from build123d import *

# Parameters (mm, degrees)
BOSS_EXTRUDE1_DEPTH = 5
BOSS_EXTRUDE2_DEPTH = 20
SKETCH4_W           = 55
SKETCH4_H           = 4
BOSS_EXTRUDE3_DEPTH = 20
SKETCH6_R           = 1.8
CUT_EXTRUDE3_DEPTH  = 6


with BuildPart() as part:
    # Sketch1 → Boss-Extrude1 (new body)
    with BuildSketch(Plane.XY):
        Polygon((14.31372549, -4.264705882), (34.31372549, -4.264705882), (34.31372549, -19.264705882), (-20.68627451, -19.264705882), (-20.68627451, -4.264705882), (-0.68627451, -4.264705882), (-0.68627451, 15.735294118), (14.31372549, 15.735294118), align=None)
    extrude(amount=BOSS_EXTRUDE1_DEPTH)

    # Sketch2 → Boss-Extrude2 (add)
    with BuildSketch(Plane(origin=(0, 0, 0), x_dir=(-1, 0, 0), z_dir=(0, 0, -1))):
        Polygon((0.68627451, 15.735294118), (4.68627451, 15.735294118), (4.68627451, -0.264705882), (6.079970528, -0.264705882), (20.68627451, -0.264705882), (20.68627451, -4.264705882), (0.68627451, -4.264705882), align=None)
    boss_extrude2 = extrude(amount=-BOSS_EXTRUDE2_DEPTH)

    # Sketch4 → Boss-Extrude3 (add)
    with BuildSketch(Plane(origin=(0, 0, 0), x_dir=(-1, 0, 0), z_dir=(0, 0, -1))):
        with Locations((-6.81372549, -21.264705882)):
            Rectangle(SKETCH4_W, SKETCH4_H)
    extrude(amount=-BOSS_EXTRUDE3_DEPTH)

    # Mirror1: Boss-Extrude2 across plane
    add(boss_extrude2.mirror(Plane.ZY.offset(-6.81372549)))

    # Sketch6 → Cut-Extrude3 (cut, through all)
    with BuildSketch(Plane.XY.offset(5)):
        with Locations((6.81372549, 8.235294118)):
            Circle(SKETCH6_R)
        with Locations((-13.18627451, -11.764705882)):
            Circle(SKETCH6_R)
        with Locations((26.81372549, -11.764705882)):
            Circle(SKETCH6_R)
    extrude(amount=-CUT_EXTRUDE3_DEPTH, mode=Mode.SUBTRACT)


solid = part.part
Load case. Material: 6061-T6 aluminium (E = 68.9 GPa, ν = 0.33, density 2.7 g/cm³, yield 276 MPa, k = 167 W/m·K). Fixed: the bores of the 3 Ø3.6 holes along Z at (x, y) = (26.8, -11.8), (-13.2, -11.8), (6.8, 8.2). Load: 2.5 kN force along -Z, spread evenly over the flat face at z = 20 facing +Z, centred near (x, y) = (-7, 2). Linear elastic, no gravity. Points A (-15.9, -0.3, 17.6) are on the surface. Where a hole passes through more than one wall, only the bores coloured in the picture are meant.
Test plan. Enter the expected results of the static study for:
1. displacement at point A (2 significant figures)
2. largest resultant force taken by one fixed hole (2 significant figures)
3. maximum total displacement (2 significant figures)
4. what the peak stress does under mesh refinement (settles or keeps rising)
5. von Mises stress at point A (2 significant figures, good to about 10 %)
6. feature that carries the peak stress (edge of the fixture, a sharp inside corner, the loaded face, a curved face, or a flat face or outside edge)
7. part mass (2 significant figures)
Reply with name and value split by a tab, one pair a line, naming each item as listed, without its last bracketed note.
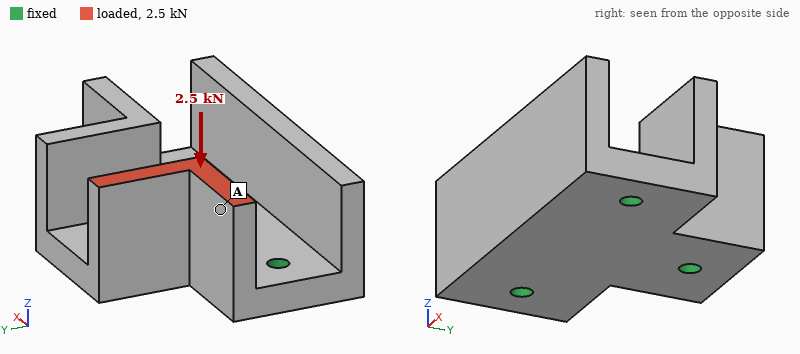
displacement at point A	46 µm
largest resultant force taken by one fixed hole	1.4 kN
maximum total displacement	57 µm
what the peak stress does under mesh refinement	keeps rising
von Mises stress at point A	16 MPa
feature that carries the peak stress	edge of the fixture
part mass	42 g
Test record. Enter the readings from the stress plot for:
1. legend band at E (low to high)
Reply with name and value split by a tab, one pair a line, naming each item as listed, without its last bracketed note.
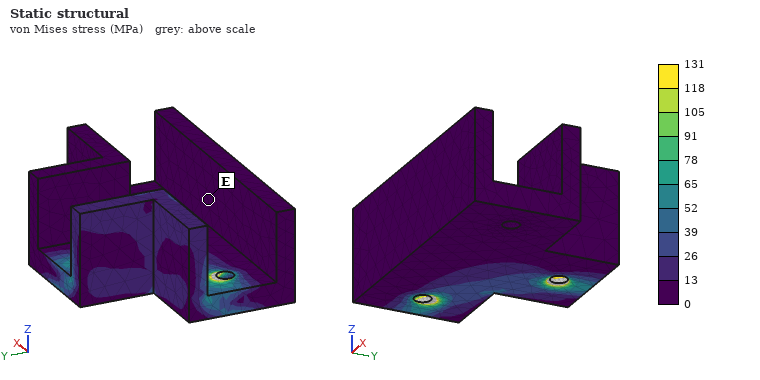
legend band at E	0 to 13 MPa
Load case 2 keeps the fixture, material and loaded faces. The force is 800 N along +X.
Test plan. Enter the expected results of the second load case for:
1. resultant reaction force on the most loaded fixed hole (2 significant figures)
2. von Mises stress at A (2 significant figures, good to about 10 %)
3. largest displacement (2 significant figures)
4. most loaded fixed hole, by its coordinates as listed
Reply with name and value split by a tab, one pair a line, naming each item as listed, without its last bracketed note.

resultant reaction force on the most loaded fixed hole	540 N
von Mises stress at A	12 MPa
largest displacement	83 µm
most loaded fixed hole, by its coordinates as listed	(-13.2, -11.8)
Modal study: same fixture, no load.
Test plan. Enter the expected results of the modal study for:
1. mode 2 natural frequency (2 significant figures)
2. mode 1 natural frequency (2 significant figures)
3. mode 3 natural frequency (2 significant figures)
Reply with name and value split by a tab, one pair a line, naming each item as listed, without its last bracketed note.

mode 2 natural frequency	9700 Hz
mode 1 natural frequency	6900 Hz
mode 3 natural frequency	10 kHz
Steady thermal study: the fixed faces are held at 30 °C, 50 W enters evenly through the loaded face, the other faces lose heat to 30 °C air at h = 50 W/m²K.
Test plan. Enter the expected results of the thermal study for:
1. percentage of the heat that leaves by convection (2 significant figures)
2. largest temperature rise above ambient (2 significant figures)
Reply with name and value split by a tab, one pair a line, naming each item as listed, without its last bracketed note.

percentage of the heat that leaves by convection	6.1 %
largest temperature rise above ambient	47 K
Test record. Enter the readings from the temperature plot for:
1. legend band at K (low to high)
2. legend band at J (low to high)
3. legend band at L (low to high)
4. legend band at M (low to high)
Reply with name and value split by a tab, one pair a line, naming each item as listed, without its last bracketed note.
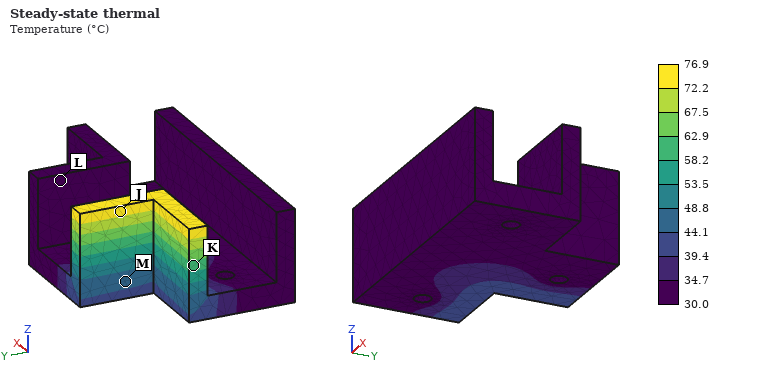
legend band at K	58.2 to 62.9 °C
legend band at J	72.2 to 76.9 °C
legend band at L	30.0 to 34.7 °C
legend band at M	44.1 to 48.8 °C
